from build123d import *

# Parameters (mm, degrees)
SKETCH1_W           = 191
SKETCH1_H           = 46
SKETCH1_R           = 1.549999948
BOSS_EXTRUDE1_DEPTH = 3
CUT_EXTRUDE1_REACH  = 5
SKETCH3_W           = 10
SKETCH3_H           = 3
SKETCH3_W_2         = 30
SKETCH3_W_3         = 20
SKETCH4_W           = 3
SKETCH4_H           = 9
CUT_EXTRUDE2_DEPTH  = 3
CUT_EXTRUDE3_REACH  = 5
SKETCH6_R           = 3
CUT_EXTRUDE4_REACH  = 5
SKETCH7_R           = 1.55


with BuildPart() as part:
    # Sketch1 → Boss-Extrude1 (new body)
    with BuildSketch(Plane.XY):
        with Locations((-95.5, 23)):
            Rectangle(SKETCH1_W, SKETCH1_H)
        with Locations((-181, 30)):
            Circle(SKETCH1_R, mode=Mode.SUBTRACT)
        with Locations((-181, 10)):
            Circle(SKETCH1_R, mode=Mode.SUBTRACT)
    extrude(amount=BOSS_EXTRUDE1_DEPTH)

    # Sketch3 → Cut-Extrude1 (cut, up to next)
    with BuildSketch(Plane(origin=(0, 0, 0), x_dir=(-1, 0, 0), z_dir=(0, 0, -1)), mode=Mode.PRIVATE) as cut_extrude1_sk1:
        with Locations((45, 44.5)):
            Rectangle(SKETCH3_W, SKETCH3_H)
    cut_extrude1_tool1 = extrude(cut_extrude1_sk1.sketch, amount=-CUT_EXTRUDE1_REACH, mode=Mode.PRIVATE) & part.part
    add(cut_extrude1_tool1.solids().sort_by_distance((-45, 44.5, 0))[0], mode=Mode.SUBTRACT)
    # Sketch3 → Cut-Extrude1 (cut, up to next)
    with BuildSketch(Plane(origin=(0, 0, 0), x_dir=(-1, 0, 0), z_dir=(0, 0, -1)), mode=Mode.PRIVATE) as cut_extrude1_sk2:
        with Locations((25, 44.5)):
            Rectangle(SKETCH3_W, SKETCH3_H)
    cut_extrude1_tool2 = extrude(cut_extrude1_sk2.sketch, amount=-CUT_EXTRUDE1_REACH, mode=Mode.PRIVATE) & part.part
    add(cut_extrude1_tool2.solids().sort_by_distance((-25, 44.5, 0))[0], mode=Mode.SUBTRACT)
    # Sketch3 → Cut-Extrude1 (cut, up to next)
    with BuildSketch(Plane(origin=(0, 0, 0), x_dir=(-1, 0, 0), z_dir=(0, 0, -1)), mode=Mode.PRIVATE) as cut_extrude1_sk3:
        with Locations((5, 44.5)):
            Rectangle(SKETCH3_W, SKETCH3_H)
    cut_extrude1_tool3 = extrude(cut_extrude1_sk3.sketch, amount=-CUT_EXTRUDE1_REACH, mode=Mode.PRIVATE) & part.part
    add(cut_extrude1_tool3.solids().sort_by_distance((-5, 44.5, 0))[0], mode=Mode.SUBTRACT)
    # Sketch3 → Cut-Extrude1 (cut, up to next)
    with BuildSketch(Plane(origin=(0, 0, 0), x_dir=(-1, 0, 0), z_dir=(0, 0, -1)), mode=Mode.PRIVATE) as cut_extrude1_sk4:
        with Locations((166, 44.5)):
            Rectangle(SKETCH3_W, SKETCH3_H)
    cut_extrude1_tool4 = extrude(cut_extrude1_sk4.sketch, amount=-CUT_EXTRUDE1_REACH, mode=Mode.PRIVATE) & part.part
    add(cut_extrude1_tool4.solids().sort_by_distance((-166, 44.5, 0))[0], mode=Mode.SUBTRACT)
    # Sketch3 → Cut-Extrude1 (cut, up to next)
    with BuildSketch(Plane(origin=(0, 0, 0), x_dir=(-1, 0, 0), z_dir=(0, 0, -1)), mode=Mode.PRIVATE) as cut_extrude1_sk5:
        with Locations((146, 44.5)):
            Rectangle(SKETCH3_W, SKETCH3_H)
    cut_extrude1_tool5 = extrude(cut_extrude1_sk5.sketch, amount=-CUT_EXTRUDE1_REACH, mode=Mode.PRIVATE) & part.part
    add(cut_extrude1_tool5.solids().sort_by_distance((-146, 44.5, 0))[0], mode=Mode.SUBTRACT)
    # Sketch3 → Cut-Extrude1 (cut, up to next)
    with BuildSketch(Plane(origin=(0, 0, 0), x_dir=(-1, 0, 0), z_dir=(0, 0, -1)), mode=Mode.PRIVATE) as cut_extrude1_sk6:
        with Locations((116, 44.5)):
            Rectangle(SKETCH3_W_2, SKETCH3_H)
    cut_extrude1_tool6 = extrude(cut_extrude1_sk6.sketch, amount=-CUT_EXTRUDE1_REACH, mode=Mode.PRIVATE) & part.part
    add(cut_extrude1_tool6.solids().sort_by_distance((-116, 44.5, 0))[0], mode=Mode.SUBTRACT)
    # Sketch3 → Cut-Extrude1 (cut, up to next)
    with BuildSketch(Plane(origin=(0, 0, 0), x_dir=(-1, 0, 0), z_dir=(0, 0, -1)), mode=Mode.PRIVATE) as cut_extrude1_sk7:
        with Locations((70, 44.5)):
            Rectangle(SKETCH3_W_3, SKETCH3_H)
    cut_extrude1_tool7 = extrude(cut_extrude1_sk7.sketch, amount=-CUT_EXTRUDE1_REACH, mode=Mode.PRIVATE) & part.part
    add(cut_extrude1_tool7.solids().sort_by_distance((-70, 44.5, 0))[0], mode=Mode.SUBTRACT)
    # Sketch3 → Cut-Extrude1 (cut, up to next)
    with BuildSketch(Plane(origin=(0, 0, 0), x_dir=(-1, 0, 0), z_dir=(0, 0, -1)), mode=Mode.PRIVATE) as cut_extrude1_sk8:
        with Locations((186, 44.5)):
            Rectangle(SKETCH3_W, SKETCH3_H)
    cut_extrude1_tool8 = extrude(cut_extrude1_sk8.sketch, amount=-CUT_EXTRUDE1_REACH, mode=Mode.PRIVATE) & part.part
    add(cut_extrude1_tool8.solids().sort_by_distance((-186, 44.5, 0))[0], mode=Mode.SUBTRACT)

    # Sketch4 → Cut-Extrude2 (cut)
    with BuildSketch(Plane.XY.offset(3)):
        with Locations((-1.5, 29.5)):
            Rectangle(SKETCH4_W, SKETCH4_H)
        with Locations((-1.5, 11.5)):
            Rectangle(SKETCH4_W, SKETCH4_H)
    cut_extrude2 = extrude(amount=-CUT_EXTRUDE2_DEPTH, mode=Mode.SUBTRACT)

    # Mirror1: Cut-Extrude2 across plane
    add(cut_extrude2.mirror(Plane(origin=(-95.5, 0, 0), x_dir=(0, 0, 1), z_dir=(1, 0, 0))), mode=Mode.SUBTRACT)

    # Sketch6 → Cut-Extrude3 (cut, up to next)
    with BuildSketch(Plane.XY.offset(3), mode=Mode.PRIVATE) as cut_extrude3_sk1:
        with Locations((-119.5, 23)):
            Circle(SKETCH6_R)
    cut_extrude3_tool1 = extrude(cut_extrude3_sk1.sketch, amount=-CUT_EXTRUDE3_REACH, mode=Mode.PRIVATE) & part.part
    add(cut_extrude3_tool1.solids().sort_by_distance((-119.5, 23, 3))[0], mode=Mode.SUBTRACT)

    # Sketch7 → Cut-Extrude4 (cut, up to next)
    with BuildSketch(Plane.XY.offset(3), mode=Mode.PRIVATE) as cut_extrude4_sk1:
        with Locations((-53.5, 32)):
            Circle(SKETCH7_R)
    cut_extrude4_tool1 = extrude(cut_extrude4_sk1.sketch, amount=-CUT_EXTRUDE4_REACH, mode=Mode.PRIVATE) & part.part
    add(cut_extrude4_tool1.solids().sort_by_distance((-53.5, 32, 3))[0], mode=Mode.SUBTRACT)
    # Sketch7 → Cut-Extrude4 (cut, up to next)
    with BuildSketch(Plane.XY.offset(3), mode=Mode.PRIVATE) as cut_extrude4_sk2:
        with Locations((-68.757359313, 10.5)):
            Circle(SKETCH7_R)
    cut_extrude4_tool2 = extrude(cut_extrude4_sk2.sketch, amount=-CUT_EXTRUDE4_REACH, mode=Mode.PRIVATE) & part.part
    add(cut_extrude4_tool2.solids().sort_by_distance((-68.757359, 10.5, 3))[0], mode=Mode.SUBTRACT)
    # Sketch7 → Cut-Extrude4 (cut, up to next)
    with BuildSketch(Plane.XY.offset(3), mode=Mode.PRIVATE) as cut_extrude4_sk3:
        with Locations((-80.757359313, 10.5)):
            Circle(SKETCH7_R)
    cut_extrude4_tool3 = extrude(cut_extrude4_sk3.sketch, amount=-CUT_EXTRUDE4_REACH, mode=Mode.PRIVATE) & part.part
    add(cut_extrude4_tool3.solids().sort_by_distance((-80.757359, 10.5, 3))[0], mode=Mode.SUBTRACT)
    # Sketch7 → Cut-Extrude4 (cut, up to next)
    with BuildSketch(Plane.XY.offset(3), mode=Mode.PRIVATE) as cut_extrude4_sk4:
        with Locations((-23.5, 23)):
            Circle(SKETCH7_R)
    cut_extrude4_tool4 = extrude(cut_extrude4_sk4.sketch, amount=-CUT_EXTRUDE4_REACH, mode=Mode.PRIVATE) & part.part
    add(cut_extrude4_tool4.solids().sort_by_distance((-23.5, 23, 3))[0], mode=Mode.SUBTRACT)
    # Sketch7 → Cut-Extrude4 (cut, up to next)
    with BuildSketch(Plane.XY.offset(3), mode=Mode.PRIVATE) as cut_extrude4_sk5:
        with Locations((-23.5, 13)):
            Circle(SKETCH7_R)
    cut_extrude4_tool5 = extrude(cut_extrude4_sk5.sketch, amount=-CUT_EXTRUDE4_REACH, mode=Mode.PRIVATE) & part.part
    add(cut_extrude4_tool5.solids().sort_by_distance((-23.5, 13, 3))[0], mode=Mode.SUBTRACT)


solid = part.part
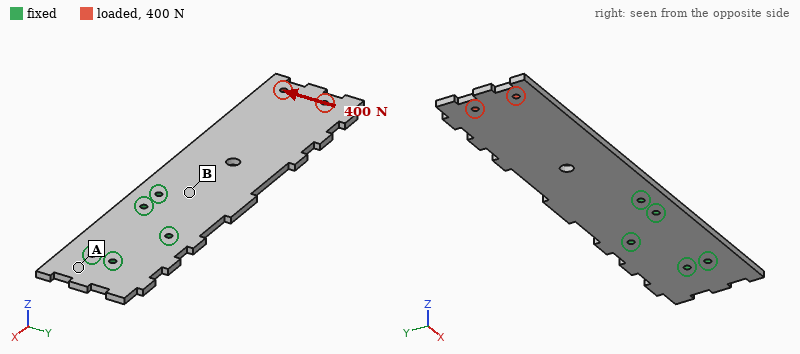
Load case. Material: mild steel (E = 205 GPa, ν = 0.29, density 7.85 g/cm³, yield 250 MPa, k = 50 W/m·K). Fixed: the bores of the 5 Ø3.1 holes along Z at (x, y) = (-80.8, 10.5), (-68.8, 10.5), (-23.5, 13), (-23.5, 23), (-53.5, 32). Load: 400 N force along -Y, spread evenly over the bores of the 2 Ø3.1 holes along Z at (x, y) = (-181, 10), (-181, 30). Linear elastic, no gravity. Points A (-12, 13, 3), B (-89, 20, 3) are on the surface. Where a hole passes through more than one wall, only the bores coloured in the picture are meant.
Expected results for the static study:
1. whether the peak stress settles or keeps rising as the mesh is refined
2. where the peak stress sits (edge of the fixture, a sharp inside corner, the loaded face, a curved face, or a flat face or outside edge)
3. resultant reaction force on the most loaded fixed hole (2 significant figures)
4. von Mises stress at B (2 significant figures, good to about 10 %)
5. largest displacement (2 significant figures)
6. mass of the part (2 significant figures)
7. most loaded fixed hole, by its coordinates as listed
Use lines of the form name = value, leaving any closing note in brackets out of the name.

whether the peak stress settles or keeps rising as the mesh is refined = keeps rising
where the peak stress sits = edge of the fixture
resultant reaction force on the most loaded fixed hole = 1.3 kN
von Mises stress at B = 12 MPa
largest displacement = 61 µm
mass of the part = 190 g
most loaded fixed hole, by its coordinates as listed = (-80.8, 10.5)
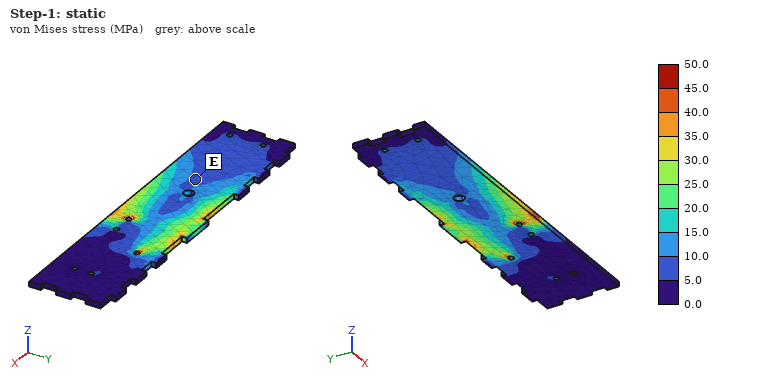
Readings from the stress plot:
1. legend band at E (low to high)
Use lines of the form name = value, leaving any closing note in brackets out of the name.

legend band at E = 5.0 to 10.0 MPa
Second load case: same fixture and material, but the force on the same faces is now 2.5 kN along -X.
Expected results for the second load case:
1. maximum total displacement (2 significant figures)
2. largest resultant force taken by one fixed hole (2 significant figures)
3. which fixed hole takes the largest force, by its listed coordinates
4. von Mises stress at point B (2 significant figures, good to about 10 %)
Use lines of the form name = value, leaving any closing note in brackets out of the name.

maximum total displacement = 13 µm
largest resultant force taken by one fixed hole = 1.2 kN
which fixed hole takes the largest force, by its listed coordinates = (-80.8, 10.5)
von Mises stress at point B = 18 MPa
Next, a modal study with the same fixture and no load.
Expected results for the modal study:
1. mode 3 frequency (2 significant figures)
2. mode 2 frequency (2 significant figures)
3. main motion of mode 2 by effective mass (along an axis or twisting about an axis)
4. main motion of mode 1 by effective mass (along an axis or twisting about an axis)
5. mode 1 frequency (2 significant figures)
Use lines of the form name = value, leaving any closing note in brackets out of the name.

mode 3 frequency = 1200 Hz
mode 2 frequency = 900 Hz
main motion of mode 2 by effective mass = twisting about X
main motion of mode 1 by effective mass = along Z
mode 1 frequency = 200 Hz
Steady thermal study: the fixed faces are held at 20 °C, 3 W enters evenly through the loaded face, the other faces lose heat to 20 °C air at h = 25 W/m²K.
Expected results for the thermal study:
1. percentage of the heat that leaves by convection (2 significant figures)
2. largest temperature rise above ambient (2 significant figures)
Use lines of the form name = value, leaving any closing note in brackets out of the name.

percentage of the heat that leaves by convection = 80 %
largest temperature rise above ambient = 22 K
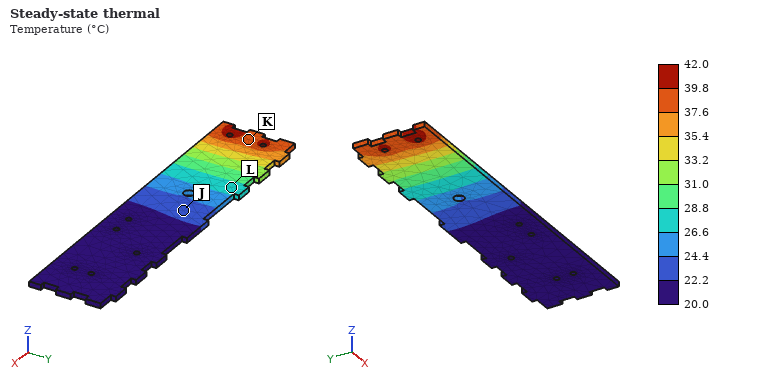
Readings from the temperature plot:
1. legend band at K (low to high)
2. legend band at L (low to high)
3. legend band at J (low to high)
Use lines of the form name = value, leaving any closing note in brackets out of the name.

legend band at K = 37.6 to 39.8 °C
legend band at L = 26.6 to 28.8 °C
legend band at J = 22.2 to 24.4 °C
